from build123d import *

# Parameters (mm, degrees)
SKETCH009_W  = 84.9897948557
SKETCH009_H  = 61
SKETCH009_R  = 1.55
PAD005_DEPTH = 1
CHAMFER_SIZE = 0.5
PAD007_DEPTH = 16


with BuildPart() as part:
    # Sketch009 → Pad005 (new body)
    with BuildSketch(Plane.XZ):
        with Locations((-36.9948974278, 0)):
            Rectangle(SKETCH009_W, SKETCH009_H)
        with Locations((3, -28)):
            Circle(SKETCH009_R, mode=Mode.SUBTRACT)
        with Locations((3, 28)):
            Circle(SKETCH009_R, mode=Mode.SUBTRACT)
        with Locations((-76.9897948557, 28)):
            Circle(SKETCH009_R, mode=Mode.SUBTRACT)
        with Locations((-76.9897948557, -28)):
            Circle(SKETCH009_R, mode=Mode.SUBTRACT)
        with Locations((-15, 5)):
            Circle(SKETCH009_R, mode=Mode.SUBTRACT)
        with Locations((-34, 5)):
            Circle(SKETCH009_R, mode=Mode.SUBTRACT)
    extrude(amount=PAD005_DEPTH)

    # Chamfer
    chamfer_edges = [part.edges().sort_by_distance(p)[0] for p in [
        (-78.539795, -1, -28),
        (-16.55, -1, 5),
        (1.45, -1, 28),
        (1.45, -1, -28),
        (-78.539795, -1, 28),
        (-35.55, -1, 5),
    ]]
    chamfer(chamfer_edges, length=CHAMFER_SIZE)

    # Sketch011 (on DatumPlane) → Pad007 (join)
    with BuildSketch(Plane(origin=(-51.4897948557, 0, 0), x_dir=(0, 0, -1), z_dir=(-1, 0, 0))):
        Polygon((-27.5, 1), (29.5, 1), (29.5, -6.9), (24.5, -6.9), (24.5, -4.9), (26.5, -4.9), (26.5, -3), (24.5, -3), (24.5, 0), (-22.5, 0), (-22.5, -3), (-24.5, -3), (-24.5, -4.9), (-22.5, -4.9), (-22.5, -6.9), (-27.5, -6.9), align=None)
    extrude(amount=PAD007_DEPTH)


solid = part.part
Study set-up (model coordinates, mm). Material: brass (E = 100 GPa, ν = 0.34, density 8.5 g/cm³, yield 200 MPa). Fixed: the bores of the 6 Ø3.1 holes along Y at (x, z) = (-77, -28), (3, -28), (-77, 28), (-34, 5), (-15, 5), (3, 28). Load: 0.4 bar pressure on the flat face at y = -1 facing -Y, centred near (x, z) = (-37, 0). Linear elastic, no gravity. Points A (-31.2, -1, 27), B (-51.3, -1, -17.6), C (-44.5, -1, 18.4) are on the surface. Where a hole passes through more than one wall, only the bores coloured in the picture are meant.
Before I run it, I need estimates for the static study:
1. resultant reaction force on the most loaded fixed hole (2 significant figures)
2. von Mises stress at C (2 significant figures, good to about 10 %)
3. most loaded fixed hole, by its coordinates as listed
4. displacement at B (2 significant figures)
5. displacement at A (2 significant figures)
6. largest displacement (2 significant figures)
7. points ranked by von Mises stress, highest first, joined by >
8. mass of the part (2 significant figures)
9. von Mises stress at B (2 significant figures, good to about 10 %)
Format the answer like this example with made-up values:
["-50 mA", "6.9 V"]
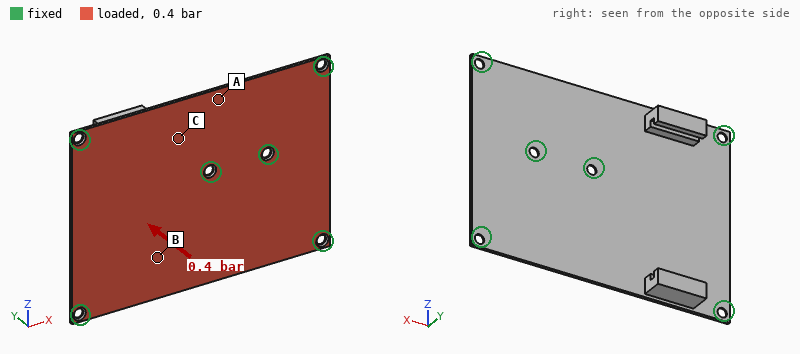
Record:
["83 N", "25 MPa", "(-34, 5)", "0.18 mm", "0.089 mm", "0.28 mm", "B > C > A", "52 g", "43 MPa"]
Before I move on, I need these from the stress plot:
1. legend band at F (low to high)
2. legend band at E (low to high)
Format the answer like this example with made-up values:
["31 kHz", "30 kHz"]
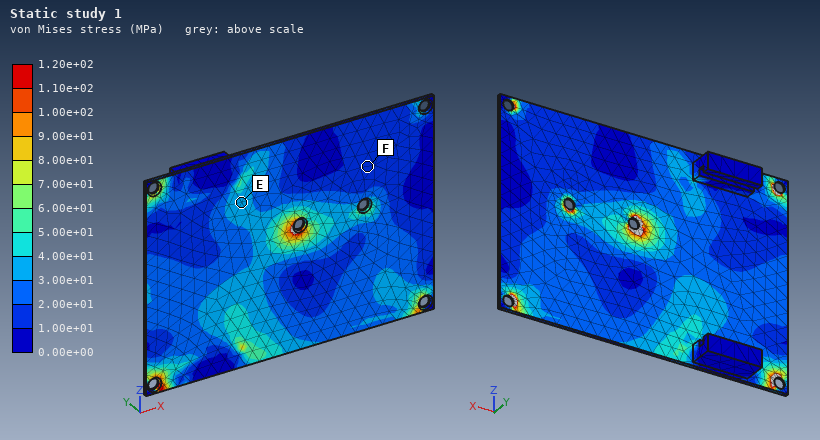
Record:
["1.00e+01 to 2.00e+01 MPa", "3.00e+01 to 4.00e+01 MPa"]
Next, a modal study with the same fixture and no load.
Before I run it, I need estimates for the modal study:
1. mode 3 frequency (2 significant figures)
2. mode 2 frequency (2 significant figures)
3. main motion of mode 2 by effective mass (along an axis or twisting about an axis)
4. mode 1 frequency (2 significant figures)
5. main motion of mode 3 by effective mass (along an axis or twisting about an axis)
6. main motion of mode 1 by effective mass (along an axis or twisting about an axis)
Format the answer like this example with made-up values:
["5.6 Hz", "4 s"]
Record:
["1100 Hz", "1000 Hz", "along Y", "720 Hz", "along Y", "along Y"]
